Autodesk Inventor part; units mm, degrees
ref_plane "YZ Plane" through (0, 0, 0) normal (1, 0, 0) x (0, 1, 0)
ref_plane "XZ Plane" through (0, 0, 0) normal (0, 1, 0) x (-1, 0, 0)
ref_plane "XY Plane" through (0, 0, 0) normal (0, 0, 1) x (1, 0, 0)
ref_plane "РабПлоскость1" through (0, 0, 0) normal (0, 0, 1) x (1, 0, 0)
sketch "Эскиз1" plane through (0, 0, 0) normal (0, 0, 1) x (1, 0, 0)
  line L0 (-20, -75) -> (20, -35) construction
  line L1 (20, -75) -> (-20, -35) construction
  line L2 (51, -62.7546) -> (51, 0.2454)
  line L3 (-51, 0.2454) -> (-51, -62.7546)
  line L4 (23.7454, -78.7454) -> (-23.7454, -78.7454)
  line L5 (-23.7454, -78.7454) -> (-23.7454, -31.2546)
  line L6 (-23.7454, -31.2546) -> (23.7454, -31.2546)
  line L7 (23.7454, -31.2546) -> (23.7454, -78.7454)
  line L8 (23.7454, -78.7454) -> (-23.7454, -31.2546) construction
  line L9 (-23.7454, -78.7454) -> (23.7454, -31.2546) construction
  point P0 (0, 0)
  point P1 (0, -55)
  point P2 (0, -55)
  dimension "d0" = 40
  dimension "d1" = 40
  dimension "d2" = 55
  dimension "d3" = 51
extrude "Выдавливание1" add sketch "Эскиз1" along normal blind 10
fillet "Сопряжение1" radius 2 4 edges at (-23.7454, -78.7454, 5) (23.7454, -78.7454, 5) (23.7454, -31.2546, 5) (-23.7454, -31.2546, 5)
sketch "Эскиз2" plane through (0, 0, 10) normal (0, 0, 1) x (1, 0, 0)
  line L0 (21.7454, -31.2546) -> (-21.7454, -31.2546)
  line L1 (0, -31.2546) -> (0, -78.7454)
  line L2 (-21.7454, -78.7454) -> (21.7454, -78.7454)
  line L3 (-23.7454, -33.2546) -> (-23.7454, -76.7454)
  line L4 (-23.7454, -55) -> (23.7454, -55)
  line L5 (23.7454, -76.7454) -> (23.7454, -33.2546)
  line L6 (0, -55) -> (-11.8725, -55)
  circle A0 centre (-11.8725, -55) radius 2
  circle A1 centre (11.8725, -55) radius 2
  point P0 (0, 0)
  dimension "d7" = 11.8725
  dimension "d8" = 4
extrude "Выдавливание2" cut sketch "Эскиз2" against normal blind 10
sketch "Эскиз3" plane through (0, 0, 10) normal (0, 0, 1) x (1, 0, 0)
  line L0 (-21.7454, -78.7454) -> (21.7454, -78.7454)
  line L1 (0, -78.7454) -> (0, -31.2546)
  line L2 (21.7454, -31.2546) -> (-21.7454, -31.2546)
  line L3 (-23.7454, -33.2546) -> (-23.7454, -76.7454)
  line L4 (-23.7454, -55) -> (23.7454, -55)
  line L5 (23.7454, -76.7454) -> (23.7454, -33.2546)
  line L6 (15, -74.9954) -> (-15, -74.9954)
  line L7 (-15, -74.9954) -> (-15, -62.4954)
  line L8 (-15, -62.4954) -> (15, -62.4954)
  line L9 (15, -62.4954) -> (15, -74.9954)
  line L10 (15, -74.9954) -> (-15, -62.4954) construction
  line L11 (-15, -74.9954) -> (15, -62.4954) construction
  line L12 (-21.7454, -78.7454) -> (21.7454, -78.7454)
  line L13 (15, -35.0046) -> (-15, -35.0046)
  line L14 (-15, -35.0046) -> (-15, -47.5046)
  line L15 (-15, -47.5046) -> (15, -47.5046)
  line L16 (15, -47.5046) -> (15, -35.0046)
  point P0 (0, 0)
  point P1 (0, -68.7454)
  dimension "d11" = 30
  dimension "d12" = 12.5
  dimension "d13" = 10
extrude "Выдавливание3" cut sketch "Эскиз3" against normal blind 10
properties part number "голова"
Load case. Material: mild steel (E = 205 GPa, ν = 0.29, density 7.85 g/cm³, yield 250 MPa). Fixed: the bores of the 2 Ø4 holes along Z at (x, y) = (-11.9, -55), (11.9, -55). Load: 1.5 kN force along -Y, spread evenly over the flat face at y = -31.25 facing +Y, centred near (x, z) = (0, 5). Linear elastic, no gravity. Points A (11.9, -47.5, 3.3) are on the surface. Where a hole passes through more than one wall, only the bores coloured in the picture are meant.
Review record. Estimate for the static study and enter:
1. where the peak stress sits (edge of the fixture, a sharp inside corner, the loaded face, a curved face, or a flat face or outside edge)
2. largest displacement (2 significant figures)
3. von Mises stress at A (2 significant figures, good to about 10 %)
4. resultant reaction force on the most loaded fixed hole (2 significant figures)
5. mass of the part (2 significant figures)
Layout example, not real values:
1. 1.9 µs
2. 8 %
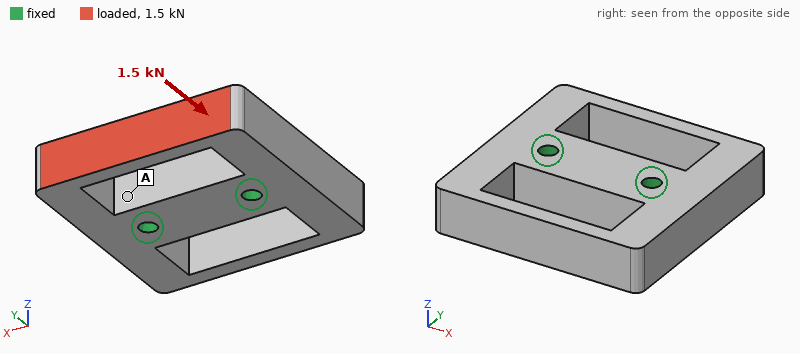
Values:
1. the loaded face
2. 18 µm
3. 13 MPa
4. 780 N
5. 120 g
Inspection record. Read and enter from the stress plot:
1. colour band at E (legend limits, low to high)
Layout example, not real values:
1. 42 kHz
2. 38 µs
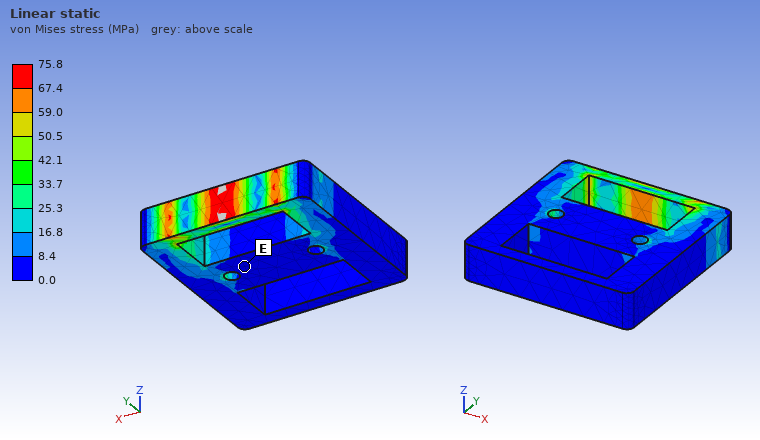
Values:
1. 0.0 to 8.4 MPa
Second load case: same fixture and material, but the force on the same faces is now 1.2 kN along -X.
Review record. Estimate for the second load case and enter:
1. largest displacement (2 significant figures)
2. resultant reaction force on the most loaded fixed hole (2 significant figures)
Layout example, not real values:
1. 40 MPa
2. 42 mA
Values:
1. 17 µm
2. 980 N
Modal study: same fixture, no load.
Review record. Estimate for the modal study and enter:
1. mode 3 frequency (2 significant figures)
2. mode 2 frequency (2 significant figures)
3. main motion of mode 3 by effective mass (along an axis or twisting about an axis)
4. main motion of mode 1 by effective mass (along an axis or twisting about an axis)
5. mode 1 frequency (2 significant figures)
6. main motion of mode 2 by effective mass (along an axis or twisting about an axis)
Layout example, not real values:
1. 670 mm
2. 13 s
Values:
1. 10 kHz
2. 8800 Hz
3. along Z
4. twisting about X
5. 8100 Hz
6. twisting about Z
